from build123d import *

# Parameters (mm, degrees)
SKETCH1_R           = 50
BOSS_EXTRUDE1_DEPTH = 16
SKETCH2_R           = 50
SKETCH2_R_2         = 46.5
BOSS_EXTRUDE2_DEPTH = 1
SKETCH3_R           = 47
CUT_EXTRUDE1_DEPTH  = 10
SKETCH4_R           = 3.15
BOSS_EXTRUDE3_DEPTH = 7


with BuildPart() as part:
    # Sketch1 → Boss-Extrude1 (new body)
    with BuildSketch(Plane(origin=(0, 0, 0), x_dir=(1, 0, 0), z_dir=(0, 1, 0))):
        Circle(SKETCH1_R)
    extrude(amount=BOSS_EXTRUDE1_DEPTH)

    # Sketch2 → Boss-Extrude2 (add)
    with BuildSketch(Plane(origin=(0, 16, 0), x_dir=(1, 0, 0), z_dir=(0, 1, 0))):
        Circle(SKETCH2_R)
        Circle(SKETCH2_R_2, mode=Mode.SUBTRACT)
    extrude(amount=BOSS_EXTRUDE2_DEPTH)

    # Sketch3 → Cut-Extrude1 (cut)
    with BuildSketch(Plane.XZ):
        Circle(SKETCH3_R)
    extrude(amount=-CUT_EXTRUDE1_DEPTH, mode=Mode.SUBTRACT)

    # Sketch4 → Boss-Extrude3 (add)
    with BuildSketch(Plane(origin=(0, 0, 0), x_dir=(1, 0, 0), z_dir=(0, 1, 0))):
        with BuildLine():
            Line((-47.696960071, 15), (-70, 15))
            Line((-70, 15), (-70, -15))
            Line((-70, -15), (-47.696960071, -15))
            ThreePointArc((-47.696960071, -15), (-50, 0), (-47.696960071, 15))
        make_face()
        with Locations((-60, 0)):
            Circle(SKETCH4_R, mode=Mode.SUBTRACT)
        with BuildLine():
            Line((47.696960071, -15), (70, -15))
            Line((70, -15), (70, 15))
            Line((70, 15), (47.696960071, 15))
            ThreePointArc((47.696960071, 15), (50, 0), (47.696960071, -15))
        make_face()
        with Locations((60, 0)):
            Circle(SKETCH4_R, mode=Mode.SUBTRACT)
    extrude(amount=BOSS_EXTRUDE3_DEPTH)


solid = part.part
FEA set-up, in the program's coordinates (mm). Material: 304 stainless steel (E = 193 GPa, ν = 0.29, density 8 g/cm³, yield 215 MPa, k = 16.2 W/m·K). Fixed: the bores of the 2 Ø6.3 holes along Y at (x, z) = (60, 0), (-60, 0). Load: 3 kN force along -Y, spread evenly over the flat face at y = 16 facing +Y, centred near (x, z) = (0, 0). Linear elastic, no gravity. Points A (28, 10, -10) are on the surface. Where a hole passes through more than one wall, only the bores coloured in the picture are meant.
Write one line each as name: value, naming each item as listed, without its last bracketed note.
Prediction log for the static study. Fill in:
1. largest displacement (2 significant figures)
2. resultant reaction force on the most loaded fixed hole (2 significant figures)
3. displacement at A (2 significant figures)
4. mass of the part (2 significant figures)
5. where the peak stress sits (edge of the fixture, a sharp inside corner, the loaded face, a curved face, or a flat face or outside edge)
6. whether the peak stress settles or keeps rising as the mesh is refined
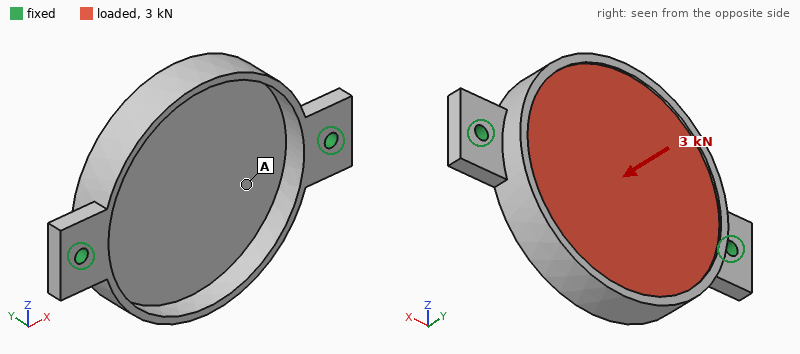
largest displacement: 42 µm
resultant reaction force on the most loaded fixed hole: 3.0 kN
displacement at A: 23 µm
mass of the part: 520 g
where the peak stress sits: edge of the fixture
whether the peak stress settles or keeps rising as the mesh is refined: keeps rising
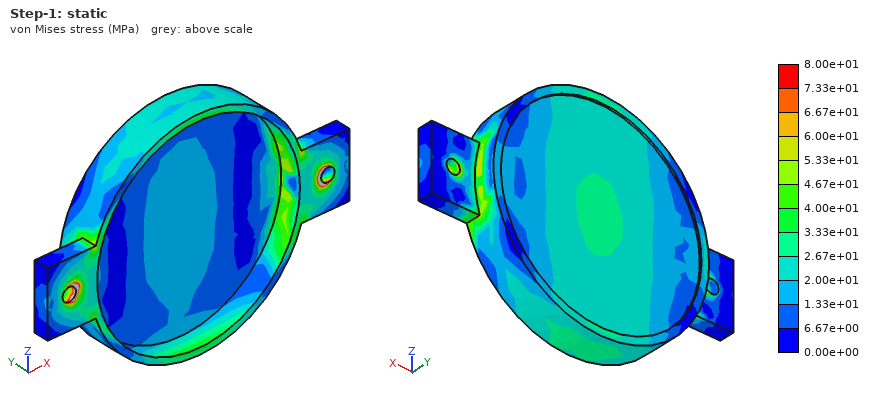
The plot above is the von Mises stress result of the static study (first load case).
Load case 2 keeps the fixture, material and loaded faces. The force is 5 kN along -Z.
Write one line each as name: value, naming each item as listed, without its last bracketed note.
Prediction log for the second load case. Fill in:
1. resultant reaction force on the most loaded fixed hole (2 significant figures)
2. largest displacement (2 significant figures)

resultant reaction force on the most loaded fixed hole: 2.5 kN
largest displacement: 0.12 mm
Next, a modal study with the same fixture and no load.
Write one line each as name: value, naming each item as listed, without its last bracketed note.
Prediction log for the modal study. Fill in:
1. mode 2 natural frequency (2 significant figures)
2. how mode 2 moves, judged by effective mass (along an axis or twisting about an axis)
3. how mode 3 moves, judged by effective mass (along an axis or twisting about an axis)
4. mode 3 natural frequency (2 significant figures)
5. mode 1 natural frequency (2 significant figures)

mode 2 natural frequency: 2400 Hz
how mode 2 moves, judged by effective mass: along Y
how mode 3 moves, judged by effective mass: along X
mode 3 natural frequency: 4100 Hz
mode 1 natural frequency: 1400 Hz
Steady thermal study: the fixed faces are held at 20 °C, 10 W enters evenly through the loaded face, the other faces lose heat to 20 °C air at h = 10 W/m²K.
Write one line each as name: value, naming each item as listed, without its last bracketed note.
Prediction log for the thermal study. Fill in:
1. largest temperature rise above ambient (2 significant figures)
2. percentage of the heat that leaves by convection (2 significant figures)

largest temperature rise above ambient: 32 K
percentage of the heat that leaves by convection: 46 %
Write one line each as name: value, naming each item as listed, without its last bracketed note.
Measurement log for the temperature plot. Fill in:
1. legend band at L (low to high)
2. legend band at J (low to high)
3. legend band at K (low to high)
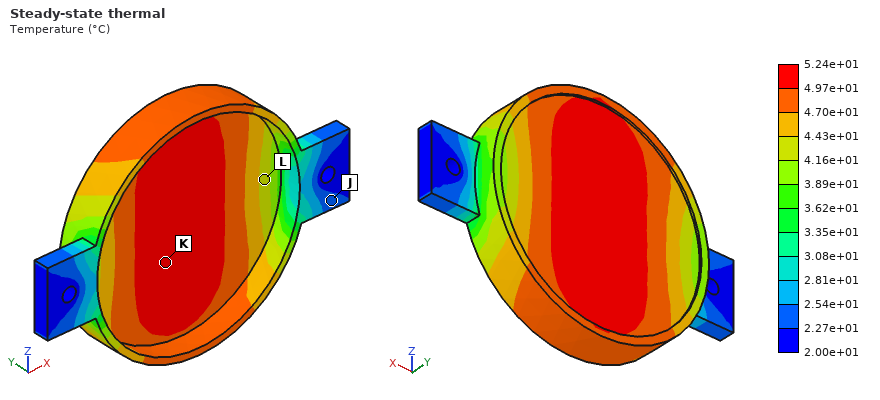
legend band at L: 4.16e+01 to 4.43e+01 °C
legend band at J: 2.27e+01 to 2.54e+01 °C
legend band at K: 4.97e+01 to 5.24e+01 °C
